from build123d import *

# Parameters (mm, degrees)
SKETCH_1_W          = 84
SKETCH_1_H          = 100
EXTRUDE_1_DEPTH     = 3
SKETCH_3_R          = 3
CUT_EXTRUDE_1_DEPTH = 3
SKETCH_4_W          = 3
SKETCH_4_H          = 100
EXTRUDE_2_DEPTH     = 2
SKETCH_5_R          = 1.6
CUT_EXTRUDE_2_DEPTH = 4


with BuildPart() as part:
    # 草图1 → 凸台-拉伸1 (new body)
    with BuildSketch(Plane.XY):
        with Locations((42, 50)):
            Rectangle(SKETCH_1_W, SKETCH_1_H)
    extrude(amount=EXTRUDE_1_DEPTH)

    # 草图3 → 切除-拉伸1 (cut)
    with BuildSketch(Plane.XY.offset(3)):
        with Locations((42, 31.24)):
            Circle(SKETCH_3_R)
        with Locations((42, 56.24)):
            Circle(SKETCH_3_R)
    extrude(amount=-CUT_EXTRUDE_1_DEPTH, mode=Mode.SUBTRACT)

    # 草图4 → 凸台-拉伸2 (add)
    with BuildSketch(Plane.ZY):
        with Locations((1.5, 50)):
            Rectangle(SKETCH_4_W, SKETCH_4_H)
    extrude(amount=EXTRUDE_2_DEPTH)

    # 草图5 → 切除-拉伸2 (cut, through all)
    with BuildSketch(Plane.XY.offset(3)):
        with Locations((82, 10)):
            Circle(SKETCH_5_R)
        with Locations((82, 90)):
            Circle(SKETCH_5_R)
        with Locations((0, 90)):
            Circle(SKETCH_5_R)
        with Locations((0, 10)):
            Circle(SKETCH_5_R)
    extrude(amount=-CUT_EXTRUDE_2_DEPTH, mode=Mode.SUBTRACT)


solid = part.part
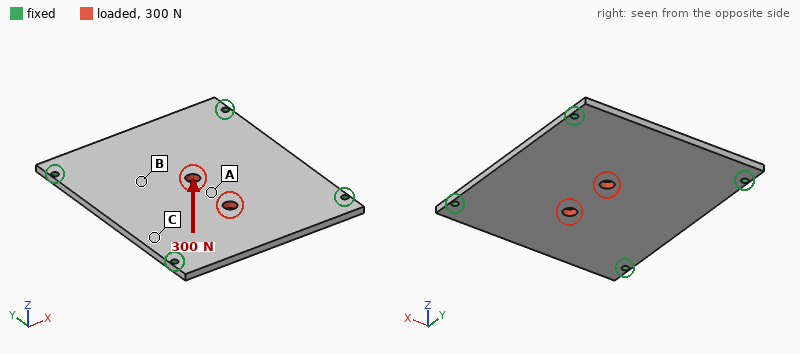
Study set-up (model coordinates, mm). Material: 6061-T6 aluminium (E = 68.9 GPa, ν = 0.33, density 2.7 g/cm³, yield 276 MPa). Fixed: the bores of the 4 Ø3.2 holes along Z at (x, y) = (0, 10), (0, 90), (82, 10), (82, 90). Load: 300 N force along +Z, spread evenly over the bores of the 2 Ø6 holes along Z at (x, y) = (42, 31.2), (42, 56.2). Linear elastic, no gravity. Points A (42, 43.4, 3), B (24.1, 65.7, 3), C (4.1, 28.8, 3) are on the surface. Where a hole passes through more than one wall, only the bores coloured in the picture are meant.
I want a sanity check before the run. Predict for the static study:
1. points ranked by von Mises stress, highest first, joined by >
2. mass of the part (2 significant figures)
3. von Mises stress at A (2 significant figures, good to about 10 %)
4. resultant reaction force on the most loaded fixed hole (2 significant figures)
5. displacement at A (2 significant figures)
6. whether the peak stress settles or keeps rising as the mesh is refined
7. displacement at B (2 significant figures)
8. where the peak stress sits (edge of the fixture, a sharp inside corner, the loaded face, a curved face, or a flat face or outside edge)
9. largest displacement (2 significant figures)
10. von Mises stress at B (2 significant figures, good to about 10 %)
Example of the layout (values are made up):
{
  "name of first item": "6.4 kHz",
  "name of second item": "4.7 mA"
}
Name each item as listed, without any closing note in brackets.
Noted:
{
  "points ranked by von Mises stress, highest first, joined by >": "A > B > C",
  "mass of the part": "69 g",
  "von Mises stress at A": "33 MPa",
  "resultant reaction force on the most loaded fixed hole": "90 N",
  "displacement at A": "0.17 mm",
  "whether the peak stress settles or keeps rising as the mesh is refined": "keeps rising",
  "displacement at B": "0.11 mm",
  "where the peak stress sits": "edge of the fixture",
  "largest displacement": "0.18 mm",
  "von Mises stress at B": "14 MPa"
}
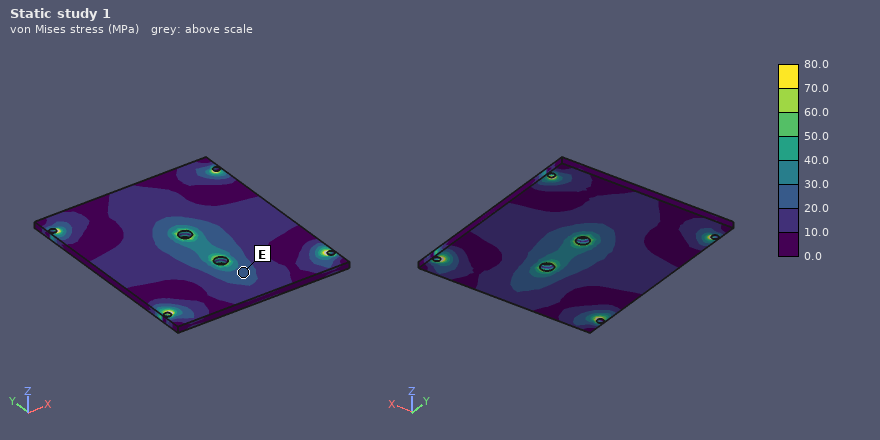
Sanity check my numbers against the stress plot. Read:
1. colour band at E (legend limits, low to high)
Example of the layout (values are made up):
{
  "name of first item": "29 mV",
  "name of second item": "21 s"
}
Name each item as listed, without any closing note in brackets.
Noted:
{
  "colour band at E": "20.0 to 30.0 MPa"
}
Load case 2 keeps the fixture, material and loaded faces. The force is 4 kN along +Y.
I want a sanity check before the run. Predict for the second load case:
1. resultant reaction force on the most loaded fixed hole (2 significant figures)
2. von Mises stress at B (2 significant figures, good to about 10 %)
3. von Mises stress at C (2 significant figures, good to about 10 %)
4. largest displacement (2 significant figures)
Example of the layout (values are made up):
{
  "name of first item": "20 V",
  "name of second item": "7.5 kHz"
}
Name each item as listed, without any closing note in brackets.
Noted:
{
  "resultant reaction force on the most loaded fixed hole": "1.1 kN",
  "von Mises stress at B": "15 MPa",
  "von Mises stress at C": "14 MPa",
  "largest displacement": "22 µm"
}
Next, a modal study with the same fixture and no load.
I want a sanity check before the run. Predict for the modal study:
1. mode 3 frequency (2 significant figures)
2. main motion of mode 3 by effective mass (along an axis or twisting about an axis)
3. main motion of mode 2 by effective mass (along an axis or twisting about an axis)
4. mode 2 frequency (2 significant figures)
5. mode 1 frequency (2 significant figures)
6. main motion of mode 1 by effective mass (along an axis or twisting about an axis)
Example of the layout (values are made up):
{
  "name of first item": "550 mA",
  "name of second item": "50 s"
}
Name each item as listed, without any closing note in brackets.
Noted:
{
  "mode 3 frequency": "2600 Hz",
  "main motion of mode 3 by effective mass": "twisting about Y",
  "main motion of mode 2 by effective mass": "twisting about X",
  "mode 2 frequency": "2400 Hz",
  "mode 1 frequency": "1400 Hz",
  "main motion of mode 1 by effective mass": "along Z"
}
